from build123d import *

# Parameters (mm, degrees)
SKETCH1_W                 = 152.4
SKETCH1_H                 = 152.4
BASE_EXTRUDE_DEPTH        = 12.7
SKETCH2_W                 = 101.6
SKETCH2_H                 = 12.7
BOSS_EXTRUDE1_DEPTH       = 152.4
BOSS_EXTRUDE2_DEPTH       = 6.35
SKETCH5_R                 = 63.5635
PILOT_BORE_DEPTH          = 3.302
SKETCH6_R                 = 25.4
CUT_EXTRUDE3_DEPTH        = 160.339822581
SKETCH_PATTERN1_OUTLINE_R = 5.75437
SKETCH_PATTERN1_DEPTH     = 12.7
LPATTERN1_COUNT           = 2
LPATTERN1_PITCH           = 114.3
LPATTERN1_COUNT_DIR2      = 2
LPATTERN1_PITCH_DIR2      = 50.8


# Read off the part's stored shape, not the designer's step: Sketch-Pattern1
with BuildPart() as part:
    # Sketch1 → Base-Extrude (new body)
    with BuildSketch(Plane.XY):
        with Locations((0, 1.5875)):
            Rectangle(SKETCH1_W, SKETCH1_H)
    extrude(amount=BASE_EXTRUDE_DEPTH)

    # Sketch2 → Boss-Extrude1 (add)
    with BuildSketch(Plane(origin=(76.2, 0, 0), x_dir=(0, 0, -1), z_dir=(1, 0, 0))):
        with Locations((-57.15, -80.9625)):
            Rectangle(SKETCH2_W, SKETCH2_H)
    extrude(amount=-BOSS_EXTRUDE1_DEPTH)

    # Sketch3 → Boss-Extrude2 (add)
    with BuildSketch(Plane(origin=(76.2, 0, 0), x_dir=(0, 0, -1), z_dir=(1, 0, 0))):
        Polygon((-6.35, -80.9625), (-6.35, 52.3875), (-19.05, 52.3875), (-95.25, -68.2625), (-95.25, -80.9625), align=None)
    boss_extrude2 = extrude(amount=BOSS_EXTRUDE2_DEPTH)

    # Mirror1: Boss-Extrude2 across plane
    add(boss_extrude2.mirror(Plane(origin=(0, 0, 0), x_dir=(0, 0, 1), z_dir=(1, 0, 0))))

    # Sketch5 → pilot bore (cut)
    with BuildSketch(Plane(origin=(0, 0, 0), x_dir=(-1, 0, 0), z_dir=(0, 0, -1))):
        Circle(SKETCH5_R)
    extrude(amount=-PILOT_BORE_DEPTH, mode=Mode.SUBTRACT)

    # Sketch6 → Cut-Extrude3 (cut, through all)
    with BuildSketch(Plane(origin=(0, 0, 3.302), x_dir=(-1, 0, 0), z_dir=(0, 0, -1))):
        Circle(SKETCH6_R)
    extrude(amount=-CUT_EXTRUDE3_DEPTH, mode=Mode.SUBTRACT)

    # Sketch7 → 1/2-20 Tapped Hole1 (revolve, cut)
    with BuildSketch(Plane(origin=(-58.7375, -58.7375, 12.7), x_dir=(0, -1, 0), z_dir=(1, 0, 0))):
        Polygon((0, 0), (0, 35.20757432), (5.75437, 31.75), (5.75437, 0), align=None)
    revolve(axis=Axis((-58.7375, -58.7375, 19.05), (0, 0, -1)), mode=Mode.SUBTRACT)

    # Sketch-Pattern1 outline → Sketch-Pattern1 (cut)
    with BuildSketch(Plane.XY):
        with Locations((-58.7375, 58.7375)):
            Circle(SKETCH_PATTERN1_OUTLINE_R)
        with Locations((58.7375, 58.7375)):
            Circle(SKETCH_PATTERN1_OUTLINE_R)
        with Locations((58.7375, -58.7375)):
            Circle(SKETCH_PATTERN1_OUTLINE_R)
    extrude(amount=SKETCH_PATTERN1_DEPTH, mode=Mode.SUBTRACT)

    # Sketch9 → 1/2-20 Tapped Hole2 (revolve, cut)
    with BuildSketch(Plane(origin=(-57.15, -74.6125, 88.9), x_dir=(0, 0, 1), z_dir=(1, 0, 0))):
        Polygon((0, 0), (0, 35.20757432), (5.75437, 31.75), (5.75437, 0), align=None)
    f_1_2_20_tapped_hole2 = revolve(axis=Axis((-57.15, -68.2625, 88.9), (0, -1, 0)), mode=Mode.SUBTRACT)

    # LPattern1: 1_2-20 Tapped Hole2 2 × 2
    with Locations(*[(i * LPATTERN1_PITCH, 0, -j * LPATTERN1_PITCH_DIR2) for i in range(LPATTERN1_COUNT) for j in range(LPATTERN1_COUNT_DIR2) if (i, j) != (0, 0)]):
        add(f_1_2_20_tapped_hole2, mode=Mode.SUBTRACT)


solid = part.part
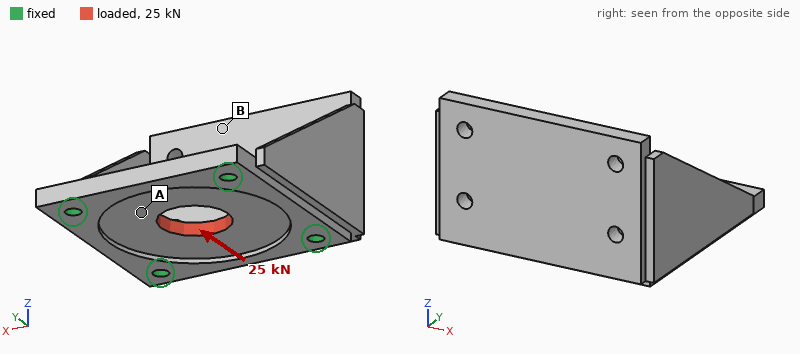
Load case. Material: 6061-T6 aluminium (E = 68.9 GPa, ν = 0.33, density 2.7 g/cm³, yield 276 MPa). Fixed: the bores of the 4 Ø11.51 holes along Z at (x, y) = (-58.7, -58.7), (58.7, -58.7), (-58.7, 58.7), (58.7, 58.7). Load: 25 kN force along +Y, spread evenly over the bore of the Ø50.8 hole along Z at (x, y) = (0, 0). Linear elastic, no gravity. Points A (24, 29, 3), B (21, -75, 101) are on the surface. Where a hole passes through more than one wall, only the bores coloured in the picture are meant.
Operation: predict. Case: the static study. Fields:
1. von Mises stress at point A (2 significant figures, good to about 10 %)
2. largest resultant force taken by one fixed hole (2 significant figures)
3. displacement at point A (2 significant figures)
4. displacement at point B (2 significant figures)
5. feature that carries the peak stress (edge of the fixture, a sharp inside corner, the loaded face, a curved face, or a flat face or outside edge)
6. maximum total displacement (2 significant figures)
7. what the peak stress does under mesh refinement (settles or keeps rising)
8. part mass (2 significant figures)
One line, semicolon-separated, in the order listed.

16 MPa; 6.8 kN; 15 µm; 9.5 µm; edge of the fixture; 23 µm; keeps rising; 1.4 kg
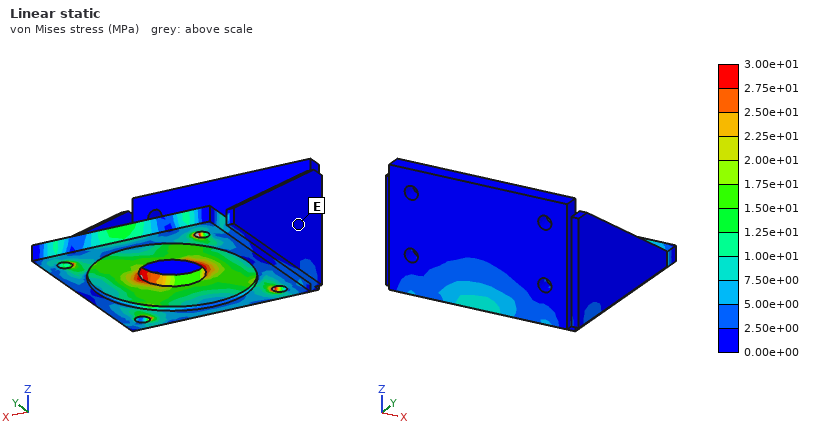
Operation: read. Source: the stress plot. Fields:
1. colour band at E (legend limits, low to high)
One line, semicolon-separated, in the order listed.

0.00e+00 to 2.50e+00 MPa
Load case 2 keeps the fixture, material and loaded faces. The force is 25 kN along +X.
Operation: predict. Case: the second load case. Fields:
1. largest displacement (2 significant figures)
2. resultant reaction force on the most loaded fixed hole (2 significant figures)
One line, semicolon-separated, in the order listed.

21 µm; 6.7 kN
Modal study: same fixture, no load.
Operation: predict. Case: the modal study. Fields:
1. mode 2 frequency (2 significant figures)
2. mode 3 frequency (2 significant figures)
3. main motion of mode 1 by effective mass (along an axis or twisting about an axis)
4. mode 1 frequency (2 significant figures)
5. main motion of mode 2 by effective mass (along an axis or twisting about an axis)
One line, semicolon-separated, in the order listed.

2700 Hz; 2900 Hz; along Y; 1400 Hz; along X
